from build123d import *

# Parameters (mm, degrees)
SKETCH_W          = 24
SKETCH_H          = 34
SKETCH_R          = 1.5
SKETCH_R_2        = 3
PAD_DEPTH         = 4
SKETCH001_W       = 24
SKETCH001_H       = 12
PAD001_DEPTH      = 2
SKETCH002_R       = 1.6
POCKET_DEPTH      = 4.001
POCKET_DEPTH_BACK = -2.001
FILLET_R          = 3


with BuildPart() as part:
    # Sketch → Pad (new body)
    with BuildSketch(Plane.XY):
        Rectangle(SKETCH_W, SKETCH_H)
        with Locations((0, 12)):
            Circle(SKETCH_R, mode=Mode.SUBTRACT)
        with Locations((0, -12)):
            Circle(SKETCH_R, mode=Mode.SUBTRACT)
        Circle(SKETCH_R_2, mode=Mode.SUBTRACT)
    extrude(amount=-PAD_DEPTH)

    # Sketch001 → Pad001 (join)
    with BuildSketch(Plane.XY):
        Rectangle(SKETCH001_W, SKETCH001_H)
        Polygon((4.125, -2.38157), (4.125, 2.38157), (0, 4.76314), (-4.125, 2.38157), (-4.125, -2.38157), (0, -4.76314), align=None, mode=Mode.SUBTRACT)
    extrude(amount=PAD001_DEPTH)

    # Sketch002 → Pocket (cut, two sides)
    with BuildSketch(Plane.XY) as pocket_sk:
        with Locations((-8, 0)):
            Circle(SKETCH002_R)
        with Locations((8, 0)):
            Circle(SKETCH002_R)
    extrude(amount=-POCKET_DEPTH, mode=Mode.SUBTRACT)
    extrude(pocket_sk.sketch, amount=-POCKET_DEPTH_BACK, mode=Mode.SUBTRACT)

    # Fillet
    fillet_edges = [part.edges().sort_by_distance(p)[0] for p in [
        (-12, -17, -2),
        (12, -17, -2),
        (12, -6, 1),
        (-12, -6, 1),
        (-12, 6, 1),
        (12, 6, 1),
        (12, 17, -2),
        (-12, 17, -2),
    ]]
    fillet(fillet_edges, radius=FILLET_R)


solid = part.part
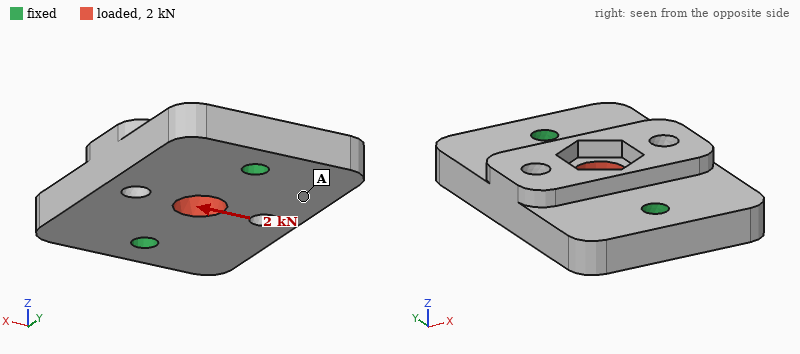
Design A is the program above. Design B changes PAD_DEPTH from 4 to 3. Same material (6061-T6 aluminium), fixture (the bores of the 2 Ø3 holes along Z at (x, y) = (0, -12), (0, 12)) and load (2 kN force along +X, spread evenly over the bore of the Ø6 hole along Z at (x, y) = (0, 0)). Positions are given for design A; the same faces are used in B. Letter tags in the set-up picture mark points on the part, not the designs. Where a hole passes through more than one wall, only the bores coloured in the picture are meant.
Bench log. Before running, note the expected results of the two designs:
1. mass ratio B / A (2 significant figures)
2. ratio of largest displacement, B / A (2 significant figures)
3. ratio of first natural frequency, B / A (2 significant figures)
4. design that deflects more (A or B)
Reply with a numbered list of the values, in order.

1. 0.78
2. 1.3
3. 0.80
4. B
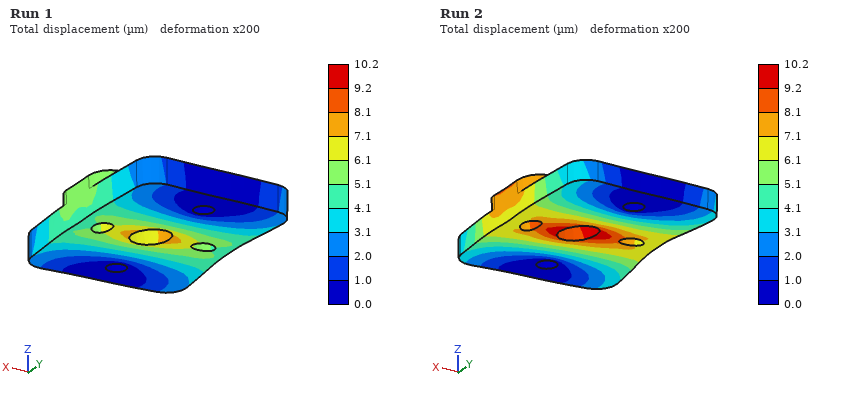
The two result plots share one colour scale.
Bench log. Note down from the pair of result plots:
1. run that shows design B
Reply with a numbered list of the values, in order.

1. Run 2
